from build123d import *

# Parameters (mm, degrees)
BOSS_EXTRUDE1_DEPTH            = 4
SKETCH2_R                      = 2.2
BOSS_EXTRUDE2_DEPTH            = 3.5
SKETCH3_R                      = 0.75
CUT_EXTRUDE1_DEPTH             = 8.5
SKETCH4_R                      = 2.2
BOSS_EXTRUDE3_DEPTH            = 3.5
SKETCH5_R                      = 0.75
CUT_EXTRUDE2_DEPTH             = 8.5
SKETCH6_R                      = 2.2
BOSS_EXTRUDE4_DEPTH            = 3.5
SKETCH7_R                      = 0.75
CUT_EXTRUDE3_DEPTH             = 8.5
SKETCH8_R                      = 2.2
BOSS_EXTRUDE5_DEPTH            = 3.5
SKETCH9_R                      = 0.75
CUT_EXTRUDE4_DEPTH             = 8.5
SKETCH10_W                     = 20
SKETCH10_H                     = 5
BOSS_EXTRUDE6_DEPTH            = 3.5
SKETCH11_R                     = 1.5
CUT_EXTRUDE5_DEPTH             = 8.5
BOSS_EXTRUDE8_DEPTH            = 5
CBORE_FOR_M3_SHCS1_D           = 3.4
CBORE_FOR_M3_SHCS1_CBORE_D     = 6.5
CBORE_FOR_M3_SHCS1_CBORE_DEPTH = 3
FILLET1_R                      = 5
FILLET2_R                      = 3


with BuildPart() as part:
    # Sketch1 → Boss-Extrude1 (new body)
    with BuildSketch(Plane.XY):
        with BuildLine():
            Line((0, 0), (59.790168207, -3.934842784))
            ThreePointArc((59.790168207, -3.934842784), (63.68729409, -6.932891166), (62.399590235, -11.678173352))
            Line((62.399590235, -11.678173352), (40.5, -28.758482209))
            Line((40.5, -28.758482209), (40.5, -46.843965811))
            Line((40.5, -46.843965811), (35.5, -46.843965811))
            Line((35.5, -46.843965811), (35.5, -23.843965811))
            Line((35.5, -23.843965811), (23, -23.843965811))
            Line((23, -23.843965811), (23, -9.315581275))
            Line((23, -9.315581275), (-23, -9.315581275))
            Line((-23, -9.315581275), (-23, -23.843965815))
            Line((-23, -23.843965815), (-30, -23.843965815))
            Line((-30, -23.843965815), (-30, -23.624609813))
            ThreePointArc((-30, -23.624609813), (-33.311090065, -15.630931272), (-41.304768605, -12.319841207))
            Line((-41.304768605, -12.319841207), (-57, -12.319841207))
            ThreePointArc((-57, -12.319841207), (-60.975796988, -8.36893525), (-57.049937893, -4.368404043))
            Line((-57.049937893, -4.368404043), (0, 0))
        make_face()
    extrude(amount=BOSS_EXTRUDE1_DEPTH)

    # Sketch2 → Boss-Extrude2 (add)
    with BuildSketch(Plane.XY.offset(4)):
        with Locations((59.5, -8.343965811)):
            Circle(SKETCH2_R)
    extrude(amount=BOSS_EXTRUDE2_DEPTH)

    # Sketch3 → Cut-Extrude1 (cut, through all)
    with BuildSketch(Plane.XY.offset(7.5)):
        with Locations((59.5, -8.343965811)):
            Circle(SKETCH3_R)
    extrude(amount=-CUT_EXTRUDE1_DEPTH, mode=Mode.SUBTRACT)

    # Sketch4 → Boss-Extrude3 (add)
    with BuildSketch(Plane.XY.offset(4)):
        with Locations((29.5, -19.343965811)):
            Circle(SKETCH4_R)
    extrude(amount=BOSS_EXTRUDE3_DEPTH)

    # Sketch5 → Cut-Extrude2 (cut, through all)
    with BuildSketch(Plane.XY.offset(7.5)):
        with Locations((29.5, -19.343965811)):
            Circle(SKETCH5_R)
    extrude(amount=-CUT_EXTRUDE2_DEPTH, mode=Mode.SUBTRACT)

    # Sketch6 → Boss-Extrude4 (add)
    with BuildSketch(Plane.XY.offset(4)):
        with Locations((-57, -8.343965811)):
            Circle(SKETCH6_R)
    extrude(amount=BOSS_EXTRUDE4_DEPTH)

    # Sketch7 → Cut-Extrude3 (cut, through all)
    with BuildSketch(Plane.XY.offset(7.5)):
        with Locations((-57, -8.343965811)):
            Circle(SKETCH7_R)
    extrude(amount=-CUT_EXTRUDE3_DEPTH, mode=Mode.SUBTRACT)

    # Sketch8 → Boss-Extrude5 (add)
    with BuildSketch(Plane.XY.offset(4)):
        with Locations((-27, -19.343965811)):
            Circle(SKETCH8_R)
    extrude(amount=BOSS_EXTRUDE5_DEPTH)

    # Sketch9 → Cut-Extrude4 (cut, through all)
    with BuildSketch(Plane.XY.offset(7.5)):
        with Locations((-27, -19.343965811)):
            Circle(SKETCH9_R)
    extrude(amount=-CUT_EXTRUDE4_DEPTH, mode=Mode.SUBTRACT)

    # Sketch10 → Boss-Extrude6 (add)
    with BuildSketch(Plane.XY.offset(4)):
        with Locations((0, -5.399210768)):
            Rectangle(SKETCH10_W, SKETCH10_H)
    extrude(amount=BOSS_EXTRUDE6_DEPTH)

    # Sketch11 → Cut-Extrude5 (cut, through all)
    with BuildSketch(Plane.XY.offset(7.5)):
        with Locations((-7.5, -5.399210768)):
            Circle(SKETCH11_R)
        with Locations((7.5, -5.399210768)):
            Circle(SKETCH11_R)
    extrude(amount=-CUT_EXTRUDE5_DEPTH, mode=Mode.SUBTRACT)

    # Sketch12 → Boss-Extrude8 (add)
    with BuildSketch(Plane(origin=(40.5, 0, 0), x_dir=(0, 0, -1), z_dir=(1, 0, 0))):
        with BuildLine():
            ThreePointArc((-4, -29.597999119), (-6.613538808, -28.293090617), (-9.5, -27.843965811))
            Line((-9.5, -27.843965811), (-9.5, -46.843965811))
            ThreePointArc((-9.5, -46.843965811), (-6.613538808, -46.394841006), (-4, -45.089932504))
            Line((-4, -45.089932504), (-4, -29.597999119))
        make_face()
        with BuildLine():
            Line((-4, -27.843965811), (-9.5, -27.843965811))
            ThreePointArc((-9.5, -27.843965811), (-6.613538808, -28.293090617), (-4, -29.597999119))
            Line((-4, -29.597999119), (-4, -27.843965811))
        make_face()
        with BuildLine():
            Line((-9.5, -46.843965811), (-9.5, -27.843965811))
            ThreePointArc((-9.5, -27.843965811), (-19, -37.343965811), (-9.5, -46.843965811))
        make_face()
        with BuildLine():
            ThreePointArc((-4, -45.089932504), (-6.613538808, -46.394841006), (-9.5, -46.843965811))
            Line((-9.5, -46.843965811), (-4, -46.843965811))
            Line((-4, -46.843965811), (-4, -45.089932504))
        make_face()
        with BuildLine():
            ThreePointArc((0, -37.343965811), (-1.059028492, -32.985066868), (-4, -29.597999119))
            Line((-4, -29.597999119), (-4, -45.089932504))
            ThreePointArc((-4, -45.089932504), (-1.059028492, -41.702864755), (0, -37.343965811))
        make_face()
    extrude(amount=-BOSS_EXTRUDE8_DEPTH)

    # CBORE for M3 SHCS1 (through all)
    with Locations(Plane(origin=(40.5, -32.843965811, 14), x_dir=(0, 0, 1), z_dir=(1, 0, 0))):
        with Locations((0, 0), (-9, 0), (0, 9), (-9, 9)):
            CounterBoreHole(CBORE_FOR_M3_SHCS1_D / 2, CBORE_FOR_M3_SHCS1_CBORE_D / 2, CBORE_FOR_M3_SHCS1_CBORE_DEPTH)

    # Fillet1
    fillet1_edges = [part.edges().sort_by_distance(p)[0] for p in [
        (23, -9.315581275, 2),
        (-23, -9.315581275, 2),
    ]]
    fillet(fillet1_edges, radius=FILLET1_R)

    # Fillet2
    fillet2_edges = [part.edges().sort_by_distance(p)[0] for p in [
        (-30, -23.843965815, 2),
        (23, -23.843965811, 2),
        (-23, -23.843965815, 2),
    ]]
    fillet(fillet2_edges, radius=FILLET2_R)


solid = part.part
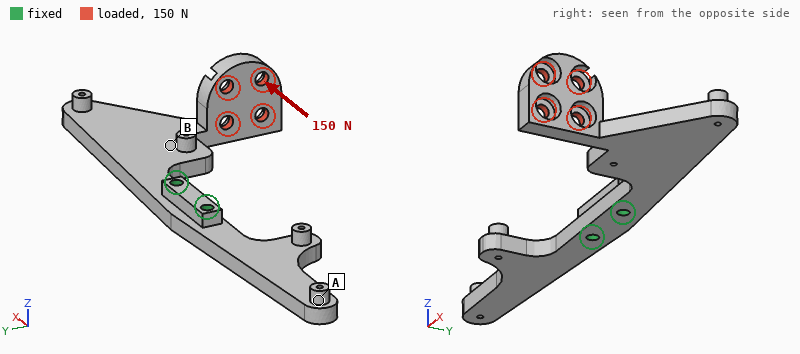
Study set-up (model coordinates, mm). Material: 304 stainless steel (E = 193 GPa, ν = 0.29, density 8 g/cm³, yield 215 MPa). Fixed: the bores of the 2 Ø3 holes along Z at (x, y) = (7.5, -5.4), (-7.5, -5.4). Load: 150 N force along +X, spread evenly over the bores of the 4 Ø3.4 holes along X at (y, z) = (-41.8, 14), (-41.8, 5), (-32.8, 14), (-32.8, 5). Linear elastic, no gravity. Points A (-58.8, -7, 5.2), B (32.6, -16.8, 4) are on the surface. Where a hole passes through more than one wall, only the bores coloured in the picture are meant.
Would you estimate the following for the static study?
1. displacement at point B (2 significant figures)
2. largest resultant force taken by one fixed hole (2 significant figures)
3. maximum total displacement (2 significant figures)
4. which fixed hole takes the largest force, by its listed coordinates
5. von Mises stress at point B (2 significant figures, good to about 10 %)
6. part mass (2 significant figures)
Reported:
0.065 mm
260 N
0.22 mm
(7.5, -5.4)
30 MPa
64 g
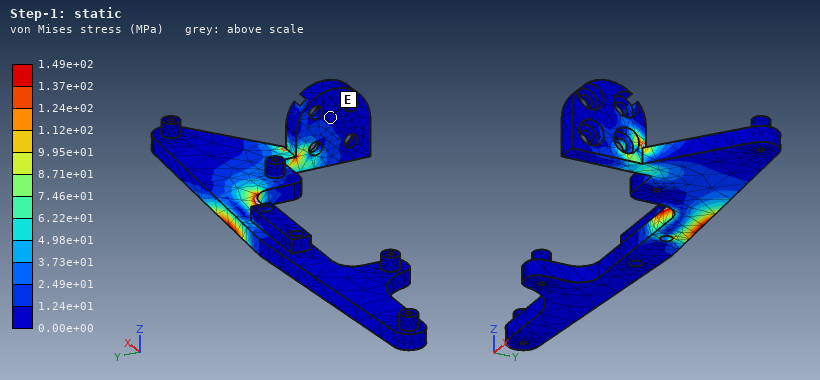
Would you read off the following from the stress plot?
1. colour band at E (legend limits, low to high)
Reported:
0.00e+00 to 1.24e+01 MPa
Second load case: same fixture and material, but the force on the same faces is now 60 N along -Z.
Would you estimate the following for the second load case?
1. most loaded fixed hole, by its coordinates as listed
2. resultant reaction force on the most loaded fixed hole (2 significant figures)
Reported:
(7.5, -5.4)
68 N
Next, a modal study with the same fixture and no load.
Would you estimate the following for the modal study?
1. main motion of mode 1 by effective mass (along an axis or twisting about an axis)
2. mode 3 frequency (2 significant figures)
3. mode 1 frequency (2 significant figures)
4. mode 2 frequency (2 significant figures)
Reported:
along Z
1100 Hz
630 Hz
1100 Hz
